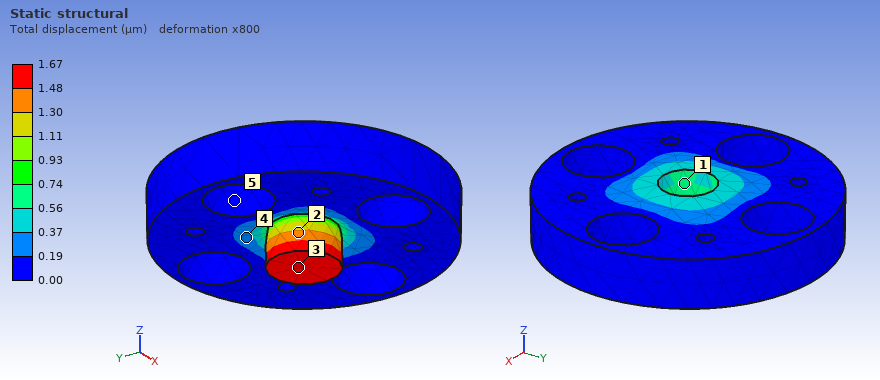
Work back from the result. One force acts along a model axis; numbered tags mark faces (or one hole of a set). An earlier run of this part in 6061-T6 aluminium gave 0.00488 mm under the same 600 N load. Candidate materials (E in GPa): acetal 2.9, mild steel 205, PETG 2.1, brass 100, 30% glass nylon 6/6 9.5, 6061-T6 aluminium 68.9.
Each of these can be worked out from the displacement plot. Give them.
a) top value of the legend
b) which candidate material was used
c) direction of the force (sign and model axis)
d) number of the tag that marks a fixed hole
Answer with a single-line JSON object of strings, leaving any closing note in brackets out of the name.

{"top value of the legend": "1.67 µm", "which candidate material was used": "mild steel", "direction of the force": "+Z", "number of the tag that marks a fixed hole": "5"}
